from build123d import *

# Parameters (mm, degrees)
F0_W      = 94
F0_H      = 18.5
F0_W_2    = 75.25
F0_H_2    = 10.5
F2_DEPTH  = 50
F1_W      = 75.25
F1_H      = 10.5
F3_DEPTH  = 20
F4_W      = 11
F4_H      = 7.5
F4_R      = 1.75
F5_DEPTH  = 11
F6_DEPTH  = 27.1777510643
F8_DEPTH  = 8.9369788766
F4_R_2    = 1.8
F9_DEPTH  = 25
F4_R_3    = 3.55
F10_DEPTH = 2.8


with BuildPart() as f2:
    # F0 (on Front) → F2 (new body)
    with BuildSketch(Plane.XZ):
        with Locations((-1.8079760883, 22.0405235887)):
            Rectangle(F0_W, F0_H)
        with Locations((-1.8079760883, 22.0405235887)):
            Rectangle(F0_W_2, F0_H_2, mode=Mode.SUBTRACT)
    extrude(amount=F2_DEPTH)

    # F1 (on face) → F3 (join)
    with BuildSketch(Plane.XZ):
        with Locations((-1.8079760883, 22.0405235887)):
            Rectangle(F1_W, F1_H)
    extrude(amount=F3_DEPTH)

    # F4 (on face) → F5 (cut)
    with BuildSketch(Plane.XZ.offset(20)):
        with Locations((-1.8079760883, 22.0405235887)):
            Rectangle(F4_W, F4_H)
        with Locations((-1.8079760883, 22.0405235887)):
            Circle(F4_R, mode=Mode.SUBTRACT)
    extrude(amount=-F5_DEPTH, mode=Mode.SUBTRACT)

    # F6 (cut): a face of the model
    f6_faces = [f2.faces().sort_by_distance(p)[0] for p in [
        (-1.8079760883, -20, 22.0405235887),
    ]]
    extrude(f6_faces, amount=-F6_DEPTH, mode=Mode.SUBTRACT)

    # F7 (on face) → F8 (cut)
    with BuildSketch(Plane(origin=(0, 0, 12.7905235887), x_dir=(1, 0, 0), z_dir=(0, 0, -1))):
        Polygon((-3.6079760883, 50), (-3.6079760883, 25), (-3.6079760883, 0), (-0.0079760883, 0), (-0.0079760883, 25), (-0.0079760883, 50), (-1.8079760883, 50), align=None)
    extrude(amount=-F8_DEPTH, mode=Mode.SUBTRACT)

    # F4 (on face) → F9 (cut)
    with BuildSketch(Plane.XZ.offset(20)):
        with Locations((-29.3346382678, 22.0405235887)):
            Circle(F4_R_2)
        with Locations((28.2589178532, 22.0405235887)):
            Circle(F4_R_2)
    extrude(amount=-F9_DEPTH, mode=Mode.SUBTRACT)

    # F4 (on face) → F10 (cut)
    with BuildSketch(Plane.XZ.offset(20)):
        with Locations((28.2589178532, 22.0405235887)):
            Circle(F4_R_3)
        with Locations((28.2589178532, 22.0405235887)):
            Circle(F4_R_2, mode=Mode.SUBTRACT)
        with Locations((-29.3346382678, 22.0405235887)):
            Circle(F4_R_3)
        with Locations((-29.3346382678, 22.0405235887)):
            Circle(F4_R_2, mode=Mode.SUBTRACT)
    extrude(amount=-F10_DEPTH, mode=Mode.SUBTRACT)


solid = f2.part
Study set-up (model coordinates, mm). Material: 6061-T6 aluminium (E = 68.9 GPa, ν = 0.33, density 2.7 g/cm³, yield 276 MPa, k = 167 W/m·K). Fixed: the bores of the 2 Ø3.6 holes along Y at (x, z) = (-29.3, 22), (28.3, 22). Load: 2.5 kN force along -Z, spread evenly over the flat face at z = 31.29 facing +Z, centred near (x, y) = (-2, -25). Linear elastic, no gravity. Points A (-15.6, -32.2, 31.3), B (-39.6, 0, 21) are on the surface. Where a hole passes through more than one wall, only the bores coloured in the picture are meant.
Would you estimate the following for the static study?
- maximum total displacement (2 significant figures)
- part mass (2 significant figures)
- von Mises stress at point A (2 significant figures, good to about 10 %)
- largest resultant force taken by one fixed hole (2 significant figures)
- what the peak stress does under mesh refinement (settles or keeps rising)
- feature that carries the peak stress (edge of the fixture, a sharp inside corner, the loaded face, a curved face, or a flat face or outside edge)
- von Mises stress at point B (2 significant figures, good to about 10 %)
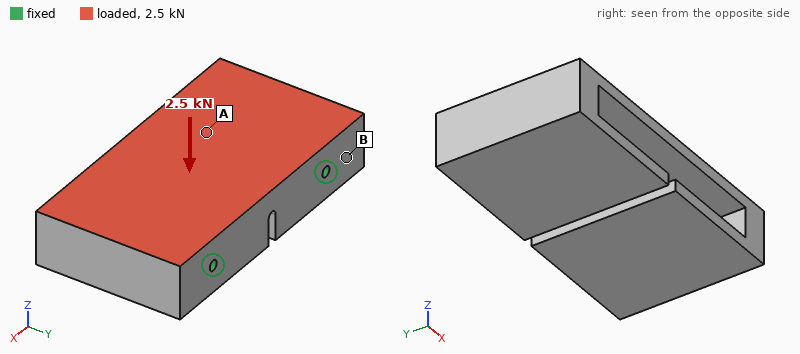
0.11 mm
160 g
15 MPa
1.4 kN
keeps rising
edge of the fixture
4.8 MPa
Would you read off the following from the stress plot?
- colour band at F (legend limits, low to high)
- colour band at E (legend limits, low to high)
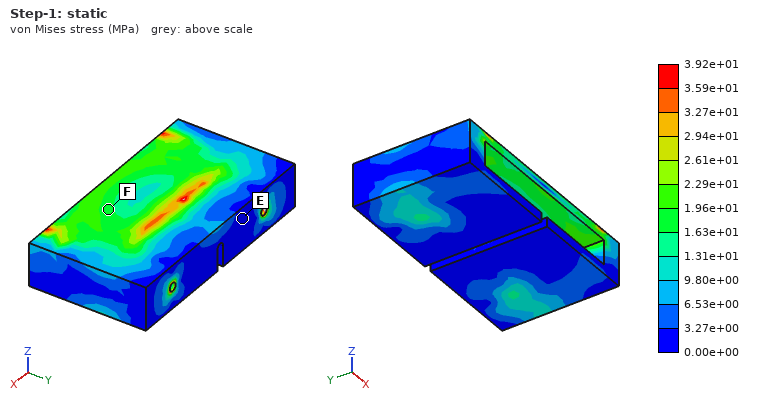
1.63e+01 to 1.96e+01 MPa
0.00e+00 to 3.27e+00 MPa
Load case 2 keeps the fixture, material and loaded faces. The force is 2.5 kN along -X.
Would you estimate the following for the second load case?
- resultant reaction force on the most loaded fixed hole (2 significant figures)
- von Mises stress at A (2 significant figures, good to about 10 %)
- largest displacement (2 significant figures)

1.4 kN
4.7 MPa
7.7 µm
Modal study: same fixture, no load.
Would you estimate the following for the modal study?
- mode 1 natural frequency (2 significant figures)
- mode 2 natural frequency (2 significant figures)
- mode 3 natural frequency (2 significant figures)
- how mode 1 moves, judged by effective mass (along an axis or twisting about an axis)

4200 Hz
4600 Hz
5400 Hz
along Z
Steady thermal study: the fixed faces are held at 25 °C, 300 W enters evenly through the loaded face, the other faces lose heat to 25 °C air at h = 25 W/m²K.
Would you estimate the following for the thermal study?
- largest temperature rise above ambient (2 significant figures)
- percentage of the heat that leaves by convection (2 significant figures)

64 K
3.3 %
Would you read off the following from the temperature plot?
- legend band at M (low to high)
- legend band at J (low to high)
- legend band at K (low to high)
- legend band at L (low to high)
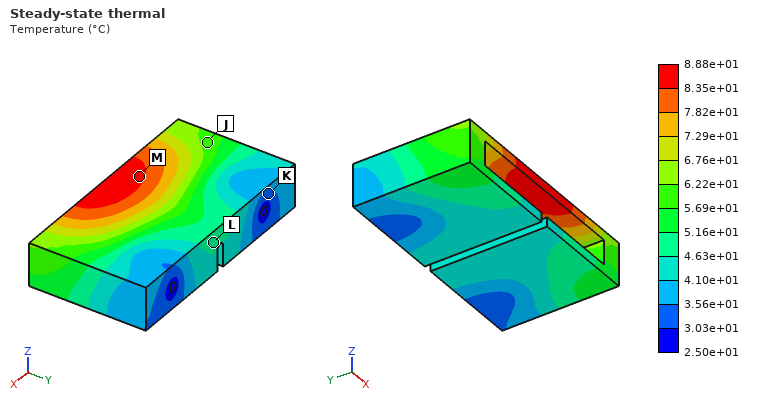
8.35e+01 to 8.88e+01 °C
5.69e+01 to 6.22e+01 °C
3.03e+01 to 3.56e+01 °C
4.63e+01 to 5.16e+01 °C
